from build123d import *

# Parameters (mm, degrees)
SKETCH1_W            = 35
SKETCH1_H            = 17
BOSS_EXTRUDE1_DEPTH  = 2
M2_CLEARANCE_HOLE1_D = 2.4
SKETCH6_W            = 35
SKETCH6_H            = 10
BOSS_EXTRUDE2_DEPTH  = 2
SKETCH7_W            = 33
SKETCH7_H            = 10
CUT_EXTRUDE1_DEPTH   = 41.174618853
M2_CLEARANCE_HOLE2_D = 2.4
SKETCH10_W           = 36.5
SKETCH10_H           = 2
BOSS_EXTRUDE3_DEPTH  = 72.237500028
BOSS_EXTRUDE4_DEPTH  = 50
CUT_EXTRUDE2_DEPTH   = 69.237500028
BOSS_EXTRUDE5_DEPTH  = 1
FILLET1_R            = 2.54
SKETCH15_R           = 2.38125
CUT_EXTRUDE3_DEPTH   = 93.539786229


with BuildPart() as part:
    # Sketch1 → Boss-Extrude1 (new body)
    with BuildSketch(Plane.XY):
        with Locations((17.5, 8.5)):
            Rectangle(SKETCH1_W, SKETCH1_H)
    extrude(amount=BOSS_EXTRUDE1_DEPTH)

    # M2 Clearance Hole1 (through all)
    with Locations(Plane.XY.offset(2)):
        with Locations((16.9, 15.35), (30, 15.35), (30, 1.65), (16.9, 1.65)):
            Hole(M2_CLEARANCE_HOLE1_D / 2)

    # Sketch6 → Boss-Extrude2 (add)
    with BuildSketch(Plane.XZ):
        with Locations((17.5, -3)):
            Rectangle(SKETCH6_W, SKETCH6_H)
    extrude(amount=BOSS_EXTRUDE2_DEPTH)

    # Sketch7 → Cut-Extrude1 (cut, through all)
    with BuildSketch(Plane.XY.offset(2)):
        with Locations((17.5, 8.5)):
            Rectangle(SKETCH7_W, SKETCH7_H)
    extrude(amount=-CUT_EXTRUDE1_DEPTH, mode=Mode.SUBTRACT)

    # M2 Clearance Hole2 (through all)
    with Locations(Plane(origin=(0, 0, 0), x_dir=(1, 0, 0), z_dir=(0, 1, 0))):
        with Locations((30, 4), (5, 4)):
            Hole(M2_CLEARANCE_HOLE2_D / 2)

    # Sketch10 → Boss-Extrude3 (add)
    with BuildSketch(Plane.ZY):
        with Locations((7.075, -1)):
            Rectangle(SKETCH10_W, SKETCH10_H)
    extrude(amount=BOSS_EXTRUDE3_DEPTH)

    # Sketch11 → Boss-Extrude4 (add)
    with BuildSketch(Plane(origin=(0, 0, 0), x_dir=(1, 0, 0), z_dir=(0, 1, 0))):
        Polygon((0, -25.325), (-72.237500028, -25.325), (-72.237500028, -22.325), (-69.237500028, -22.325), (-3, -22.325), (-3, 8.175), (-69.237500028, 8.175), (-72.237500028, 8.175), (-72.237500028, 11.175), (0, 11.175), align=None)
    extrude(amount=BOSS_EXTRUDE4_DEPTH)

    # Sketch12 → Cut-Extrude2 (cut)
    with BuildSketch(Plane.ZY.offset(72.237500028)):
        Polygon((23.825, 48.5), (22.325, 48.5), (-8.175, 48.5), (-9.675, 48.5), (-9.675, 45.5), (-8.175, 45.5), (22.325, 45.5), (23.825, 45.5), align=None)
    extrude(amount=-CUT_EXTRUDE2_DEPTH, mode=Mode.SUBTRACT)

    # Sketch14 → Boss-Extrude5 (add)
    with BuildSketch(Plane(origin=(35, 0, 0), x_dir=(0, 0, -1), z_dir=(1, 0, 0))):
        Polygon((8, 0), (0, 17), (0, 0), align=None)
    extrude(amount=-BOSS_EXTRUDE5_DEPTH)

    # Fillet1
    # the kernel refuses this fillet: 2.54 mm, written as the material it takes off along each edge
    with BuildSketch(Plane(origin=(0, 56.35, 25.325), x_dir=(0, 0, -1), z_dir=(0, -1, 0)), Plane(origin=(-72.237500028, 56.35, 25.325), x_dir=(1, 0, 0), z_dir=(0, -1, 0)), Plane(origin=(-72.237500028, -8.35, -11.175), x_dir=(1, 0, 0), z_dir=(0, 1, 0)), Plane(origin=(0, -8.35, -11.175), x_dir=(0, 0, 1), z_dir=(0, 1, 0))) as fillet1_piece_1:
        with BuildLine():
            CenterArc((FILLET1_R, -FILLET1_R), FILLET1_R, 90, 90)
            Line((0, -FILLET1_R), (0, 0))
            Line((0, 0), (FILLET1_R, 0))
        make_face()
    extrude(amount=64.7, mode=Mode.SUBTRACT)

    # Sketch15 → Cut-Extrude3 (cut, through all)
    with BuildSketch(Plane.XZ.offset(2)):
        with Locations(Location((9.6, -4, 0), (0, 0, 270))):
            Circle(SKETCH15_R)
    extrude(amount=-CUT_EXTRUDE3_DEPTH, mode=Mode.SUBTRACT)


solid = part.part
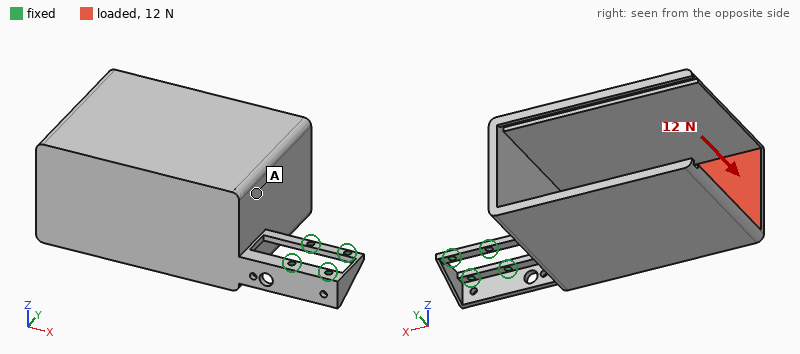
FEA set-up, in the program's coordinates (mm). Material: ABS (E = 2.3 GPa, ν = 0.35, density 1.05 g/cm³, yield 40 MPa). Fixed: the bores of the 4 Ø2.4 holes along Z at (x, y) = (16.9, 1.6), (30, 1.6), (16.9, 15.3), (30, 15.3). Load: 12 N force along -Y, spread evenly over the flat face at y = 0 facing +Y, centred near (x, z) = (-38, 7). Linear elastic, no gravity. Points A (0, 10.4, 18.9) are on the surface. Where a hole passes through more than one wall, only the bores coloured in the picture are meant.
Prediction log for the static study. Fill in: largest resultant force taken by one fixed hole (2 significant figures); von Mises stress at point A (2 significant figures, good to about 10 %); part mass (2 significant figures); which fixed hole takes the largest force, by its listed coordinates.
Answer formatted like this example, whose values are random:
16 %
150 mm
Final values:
36 N
0.82 MPa
33 g
(16.9, 15.3)
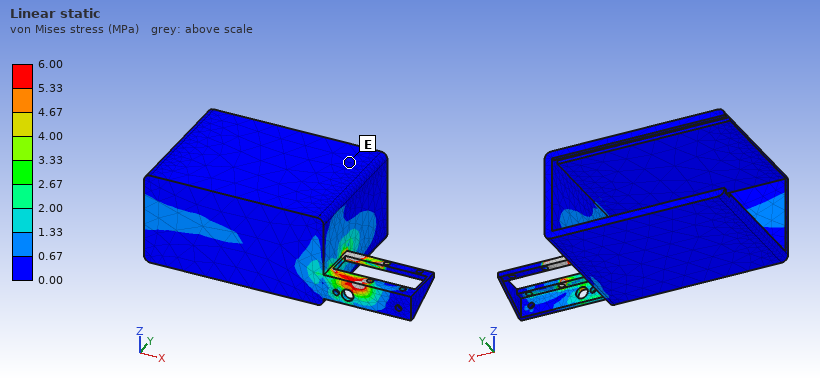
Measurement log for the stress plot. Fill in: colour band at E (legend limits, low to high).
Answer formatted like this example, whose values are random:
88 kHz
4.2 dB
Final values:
0.00 to 0.67 MPa
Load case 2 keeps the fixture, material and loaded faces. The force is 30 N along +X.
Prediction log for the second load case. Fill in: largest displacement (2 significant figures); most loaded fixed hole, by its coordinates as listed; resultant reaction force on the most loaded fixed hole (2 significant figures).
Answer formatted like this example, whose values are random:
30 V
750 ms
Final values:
1.2 mm
(16.9, 1.6)
41 N
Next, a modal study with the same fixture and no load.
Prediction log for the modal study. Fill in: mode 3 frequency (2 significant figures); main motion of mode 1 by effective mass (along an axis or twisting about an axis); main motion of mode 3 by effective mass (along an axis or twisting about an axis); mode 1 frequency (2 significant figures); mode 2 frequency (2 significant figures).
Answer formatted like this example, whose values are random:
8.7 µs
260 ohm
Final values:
160 Hz
along Z
along Y
59 Hz
100 Hz
